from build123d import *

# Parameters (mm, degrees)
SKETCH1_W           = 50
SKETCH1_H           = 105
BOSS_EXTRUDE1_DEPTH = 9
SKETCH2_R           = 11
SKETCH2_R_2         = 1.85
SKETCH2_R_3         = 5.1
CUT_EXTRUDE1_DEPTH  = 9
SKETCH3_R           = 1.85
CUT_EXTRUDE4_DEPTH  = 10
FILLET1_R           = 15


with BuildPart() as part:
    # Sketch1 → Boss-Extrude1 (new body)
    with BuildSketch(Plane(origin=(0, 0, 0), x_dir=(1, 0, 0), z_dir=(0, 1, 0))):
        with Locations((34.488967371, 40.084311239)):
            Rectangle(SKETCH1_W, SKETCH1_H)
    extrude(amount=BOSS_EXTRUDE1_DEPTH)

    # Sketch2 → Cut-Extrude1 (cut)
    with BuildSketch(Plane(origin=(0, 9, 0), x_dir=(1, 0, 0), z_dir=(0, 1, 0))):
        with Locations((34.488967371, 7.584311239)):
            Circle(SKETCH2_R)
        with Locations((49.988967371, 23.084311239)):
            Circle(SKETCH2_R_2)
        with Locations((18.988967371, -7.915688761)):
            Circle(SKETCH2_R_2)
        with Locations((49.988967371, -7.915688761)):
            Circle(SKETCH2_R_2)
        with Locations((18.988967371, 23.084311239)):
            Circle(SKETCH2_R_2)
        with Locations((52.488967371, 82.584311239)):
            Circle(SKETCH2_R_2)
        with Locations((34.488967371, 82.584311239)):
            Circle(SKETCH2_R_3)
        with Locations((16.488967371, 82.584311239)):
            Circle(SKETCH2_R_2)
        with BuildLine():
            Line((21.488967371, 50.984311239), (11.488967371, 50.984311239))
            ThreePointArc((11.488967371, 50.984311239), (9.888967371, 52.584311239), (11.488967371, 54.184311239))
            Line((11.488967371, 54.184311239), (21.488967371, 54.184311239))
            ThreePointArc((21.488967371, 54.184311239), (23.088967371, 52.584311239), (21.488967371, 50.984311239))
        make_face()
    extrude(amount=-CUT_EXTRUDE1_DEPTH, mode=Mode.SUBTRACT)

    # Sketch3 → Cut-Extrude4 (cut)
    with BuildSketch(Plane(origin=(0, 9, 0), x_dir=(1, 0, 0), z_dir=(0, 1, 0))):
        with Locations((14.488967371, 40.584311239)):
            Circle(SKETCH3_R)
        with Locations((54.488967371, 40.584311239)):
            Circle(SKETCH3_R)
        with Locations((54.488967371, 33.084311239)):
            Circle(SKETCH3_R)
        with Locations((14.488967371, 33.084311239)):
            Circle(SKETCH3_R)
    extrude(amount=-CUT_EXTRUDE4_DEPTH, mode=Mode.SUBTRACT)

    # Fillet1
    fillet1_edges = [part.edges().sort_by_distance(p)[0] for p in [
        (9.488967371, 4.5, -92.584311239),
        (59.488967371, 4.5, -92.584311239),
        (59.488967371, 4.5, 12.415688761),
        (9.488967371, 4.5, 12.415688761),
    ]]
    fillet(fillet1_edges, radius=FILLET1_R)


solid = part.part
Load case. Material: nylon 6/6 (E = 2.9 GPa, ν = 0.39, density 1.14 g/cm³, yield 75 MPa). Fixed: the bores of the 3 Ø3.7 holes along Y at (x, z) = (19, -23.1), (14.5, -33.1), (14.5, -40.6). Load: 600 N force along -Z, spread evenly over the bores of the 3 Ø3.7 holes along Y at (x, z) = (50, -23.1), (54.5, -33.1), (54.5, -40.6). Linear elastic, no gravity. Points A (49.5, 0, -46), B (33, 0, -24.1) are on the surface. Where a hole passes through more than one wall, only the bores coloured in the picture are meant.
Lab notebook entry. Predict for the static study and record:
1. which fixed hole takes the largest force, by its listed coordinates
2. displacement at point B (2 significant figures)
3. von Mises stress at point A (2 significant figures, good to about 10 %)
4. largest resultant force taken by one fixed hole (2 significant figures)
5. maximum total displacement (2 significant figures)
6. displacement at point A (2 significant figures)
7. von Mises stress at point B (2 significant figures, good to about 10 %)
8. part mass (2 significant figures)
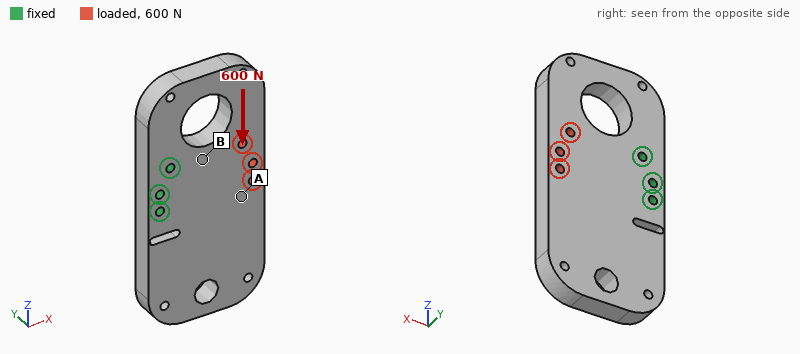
(19, -23.1)
0.085 mm
2.1 MPa
1.2 kN
0.38 mm
0.21 mm
5.2 MPa
46 g
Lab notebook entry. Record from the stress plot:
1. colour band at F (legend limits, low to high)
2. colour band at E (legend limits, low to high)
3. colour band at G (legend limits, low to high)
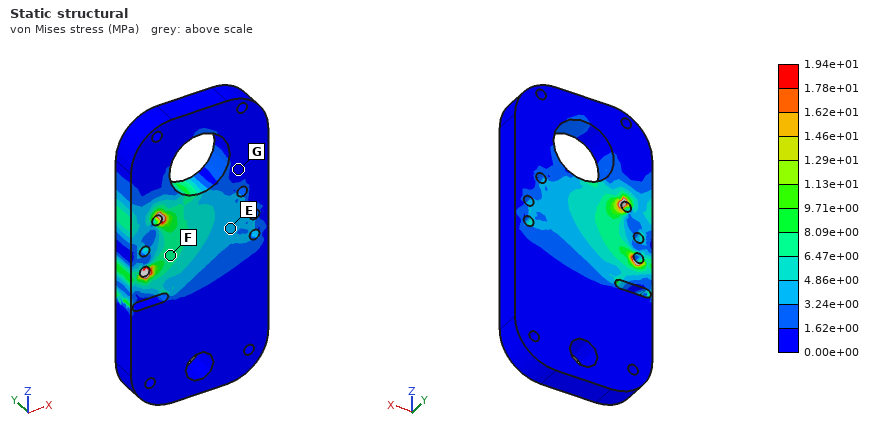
6.47e+00 to 8.09e+00 MPa
3.24e+00 to 4.86e+00 MPa
0.00e+00 to 1.62e+00 MPa
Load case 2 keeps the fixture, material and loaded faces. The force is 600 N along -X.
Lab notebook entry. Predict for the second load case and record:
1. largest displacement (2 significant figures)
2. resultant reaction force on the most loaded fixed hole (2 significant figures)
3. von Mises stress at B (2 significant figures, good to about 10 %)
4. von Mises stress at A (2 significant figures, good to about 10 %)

34 µm
240 N
2.3 MPa
1.3 MPa
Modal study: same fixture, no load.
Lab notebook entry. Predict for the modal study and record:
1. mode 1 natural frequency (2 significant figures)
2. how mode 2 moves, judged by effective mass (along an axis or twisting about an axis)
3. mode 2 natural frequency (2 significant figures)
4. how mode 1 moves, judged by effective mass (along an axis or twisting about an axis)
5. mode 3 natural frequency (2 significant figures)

550 Hz
along Y
910 Hz
along Y
1200 Hz
